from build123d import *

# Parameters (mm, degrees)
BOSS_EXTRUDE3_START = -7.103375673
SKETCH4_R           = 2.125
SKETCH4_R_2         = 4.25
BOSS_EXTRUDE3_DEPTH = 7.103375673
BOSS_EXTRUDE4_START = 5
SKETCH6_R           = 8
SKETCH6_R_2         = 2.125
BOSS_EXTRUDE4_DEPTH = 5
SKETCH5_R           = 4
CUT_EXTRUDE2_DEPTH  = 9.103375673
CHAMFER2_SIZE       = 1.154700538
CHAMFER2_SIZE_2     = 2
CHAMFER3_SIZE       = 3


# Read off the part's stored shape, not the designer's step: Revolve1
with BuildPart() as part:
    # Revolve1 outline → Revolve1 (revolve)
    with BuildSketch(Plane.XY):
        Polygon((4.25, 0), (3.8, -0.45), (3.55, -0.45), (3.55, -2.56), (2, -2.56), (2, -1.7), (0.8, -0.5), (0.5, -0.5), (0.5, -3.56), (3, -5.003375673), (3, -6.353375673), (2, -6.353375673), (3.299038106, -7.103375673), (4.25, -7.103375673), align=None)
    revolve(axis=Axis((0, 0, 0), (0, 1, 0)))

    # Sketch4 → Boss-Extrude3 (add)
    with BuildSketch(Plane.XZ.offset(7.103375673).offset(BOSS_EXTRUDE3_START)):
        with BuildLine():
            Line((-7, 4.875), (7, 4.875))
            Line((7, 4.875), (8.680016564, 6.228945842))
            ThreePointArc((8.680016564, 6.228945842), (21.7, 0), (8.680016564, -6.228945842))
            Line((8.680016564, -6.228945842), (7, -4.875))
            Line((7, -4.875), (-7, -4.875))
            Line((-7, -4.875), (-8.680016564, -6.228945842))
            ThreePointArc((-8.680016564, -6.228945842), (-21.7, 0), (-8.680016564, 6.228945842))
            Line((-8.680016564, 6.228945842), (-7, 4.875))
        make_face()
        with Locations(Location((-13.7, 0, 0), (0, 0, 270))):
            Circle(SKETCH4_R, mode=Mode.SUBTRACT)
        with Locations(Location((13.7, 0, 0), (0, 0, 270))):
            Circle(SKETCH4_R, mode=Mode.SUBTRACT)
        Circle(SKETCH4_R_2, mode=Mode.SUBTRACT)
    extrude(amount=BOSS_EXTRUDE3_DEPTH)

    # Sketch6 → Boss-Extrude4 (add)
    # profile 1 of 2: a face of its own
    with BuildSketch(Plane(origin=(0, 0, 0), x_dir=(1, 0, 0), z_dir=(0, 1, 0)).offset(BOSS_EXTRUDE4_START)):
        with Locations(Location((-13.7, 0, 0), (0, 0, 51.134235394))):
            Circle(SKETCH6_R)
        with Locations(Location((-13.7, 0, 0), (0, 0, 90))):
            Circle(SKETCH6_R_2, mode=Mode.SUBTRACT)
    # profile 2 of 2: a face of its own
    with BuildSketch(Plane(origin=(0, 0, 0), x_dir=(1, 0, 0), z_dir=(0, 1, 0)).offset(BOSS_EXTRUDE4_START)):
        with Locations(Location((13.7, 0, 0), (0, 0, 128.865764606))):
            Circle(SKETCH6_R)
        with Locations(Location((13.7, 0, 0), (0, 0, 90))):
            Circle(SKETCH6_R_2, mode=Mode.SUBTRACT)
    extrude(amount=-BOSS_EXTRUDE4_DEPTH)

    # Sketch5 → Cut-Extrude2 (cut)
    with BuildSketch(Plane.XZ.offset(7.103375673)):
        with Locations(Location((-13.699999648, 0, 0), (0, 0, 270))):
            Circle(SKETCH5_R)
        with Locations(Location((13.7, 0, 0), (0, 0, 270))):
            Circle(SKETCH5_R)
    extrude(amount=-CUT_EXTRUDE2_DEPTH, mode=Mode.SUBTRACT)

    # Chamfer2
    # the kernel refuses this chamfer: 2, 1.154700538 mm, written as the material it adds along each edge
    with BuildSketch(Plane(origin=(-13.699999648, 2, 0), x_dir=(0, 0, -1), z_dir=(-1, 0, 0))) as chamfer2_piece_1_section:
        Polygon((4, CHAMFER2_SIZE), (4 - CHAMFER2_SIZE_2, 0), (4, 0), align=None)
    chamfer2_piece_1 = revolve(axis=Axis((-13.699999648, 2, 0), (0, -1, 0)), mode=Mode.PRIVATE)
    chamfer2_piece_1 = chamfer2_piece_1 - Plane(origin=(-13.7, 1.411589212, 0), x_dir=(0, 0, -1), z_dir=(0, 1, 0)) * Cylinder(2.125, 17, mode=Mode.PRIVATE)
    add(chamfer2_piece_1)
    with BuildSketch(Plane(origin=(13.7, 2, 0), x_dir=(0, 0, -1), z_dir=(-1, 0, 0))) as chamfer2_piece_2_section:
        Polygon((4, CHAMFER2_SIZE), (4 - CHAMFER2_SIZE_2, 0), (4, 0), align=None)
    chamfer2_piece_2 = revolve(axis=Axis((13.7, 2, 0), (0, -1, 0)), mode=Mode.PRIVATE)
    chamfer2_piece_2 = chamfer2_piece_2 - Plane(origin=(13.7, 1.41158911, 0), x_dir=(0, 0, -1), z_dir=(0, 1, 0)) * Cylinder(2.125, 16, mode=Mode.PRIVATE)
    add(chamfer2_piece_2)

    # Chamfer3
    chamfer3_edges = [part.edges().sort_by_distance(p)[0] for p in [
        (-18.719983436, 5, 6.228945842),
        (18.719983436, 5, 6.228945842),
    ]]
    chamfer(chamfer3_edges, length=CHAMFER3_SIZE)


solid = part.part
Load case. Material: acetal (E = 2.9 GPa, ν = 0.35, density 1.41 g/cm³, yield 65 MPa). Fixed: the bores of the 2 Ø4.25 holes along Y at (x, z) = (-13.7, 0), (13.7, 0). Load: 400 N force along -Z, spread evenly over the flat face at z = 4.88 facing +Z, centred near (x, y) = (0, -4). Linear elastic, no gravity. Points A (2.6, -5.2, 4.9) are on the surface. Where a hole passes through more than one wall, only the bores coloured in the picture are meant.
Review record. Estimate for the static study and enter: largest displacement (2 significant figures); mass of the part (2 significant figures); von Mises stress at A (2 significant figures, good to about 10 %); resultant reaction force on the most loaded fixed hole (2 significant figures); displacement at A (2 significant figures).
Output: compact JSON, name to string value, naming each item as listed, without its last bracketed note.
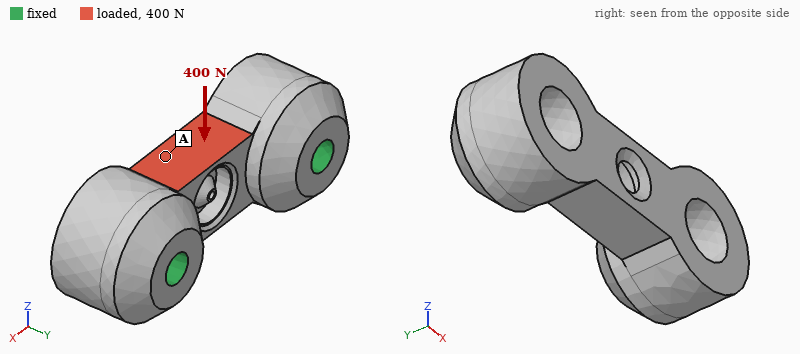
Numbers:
{"largest displacement": "0.21 mm", "mass of the part": "6.0 g", "von Mises stress at A": "8.1 MPa", "resultant reaction force on the most loaded fixed hole": "200 N", "displacement at A": "0.18 mm"}
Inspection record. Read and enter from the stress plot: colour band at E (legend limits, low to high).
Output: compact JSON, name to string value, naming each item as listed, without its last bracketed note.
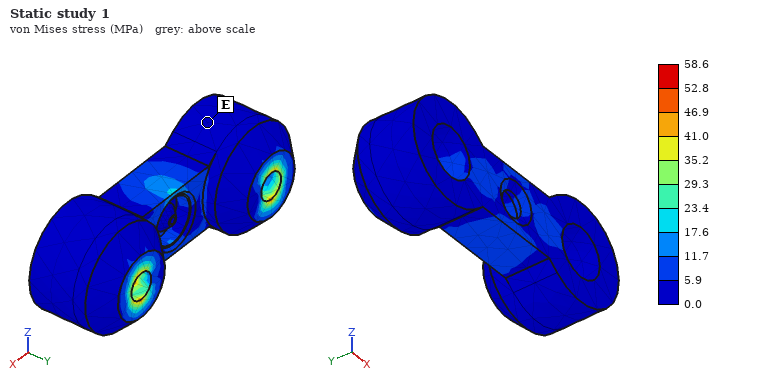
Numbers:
{"colour band at E": "0.0 to 5.9 MPa"}
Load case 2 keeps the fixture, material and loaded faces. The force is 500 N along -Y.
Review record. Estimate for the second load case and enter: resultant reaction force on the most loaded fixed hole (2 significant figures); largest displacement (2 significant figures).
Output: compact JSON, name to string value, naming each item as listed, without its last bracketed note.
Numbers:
{"resultant reaction force on the most loaded fixed hole": "340 N", "largest displacement": "0.25 mm"}
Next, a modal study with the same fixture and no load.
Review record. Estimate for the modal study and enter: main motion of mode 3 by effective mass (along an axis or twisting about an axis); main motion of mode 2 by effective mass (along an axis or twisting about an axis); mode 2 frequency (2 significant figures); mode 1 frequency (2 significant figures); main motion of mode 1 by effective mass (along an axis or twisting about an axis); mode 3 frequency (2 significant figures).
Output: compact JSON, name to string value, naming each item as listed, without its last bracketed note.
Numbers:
{"main motion of mode 3 by effective mass": "along X", "main motion of mode 2 by effective mass": "twisting about Y", "mode 2 frequency": "6100 Hz", "mode 1 frequency": "4500 Hz", "main motion of mode 1 by effective mass": "along Z", "mode 3 frequency": "7800 Hz"}
